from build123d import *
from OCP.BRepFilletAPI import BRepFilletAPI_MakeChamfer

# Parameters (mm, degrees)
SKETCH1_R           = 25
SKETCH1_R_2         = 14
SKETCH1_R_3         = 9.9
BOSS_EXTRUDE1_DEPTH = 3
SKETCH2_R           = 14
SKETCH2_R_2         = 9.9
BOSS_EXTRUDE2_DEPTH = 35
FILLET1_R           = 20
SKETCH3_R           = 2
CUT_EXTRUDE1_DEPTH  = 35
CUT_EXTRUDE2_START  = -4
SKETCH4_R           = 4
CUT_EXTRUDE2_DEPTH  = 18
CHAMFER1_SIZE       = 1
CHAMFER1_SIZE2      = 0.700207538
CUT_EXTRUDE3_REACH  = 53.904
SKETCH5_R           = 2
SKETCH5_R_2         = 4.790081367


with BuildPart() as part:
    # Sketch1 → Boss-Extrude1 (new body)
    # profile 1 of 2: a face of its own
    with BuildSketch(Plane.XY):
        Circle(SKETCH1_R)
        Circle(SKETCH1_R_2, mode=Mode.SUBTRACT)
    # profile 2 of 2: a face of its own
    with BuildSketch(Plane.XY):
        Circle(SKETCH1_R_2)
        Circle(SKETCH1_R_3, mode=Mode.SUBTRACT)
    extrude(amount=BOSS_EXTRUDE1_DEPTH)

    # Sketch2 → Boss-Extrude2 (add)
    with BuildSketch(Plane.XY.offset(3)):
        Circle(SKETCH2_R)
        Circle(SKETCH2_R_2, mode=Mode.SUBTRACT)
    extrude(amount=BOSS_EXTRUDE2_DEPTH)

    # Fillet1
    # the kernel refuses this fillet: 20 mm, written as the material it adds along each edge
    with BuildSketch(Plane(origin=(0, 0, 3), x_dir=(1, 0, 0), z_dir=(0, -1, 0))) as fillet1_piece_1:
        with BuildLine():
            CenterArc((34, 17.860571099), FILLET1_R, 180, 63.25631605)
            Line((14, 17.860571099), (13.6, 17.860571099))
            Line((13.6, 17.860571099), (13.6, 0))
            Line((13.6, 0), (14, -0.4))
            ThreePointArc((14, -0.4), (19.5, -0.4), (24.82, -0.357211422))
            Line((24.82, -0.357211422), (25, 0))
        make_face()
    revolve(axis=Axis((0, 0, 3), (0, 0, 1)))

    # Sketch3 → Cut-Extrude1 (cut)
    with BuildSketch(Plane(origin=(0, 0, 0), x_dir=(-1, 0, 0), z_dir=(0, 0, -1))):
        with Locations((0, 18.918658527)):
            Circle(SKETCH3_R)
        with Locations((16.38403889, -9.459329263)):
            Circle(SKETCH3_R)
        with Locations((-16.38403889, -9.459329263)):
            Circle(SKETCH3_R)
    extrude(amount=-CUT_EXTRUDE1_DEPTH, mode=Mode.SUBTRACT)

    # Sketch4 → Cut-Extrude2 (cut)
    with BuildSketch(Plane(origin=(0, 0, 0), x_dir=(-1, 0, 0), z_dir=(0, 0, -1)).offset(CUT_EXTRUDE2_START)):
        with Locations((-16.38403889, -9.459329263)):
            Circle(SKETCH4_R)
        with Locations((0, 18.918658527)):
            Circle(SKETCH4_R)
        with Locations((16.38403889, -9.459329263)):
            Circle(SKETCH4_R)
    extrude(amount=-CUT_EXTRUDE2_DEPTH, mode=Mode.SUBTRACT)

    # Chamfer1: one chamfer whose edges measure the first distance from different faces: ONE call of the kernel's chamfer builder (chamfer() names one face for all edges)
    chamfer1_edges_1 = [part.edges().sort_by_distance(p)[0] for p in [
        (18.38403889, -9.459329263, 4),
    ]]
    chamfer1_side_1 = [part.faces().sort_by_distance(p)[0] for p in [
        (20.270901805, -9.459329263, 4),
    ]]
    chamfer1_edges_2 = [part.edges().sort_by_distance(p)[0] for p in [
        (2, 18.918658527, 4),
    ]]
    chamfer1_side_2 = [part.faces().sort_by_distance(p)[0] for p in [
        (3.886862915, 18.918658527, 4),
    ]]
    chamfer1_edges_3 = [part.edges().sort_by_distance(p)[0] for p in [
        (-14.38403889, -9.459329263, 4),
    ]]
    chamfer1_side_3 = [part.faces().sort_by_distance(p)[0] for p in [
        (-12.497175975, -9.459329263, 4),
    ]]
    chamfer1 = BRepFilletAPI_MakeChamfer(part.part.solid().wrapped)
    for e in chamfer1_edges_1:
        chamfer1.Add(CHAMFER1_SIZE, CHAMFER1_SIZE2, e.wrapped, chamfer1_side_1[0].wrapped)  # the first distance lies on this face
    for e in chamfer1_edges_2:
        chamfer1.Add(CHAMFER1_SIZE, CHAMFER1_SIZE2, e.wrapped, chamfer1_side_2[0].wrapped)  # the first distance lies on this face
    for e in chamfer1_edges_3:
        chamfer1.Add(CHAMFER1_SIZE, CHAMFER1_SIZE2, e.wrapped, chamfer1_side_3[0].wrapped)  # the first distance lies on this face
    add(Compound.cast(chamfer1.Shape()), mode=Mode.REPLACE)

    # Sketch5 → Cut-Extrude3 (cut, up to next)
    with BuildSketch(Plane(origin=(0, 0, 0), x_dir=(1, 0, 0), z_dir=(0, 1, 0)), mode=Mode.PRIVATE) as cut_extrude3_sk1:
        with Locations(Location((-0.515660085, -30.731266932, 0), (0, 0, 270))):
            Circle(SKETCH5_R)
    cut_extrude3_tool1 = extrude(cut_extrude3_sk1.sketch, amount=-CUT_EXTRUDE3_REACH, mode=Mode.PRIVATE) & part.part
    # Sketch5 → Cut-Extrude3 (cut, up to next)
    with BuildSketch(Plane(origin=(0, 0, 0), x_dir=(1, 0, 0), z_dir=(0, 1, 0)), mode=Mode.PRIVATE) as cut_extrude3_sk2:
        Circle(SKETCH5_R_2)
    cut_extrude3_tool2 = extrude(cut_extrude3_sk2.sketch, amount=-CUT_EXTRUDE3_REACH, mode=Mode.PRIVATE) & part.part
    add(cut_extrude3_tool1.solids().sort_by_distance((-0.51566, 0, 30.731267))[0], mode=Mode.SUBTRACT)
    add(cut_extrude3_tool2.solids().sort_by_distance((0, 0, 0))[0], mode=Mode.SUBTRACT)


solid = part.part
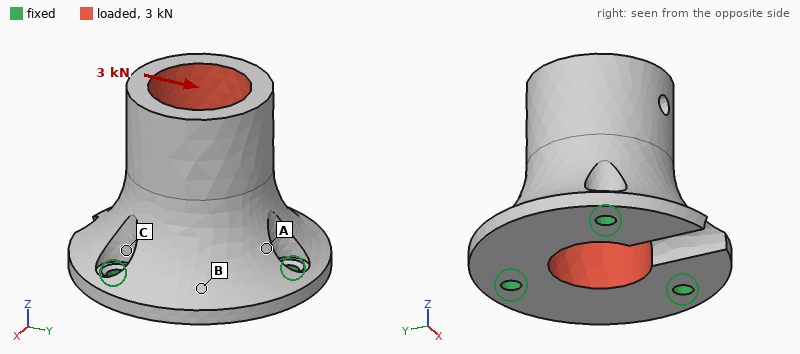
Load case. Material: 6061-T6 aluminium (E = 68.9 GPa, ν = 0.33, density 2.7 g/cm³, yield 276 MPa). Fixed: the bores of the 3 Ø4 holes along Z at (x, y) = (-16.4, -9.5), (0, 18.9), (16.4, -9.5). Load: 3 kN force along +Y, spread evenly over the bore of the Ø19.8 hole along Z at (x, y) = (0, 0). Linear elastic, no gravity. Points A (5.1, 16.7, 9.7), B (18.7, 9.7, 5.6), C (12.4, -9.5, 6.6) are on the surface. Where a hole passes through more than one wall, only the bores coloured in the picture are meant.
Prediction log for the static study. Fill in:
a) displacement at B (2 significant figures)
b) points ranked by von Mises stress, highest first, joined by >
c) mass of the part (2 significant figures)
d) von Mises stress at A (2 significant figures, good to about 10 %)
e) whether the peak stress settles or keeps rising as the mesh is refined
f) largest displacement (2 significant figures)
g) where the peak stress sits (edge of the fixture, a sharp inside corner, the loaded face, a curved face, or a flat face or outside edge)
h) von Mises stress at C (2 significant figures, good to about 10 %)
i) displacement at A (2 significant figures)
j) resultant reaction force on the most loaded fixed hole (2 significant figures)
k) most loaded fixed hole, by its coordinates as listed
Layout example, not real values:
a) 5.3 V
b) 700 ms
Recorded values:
a) 8.0 µm
b) A > C > B
c) 55 g
d) 38 MPa
e) keeps rising
f) 34 µm
g) edge of the fixture
h) 22 MPa
i) 8.5 µm
j) 2.2 kN
k) (0, 18.9)
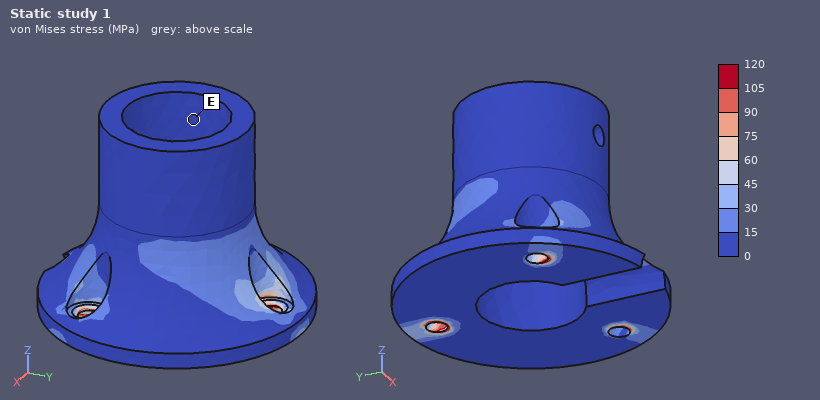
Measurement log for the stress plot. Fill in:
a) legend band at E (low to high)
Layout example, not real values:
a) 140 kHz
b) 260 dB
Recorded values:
a) 0 to 15 MPa
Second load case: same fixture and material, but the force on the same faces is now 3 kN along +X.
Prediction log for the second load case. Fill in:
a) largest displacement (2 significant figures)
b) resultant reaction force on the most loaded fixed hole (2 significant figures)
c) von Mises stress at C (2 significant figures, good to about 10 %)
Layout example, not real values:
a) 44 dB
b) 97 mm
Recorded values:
a) 33 µm
b) 2.0 kN
c) 28 MPa
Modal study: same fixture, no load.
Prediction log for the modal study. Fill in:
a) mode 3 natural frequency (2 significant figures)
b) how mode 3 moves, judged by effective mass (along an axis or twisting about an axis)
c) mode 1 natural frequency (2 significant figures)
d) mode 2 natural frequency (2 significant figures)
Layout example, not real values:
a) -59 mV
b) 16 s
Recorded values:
a) 16 kHz
b) along Z
c) 9500 Hz
d) 9600 Hz
